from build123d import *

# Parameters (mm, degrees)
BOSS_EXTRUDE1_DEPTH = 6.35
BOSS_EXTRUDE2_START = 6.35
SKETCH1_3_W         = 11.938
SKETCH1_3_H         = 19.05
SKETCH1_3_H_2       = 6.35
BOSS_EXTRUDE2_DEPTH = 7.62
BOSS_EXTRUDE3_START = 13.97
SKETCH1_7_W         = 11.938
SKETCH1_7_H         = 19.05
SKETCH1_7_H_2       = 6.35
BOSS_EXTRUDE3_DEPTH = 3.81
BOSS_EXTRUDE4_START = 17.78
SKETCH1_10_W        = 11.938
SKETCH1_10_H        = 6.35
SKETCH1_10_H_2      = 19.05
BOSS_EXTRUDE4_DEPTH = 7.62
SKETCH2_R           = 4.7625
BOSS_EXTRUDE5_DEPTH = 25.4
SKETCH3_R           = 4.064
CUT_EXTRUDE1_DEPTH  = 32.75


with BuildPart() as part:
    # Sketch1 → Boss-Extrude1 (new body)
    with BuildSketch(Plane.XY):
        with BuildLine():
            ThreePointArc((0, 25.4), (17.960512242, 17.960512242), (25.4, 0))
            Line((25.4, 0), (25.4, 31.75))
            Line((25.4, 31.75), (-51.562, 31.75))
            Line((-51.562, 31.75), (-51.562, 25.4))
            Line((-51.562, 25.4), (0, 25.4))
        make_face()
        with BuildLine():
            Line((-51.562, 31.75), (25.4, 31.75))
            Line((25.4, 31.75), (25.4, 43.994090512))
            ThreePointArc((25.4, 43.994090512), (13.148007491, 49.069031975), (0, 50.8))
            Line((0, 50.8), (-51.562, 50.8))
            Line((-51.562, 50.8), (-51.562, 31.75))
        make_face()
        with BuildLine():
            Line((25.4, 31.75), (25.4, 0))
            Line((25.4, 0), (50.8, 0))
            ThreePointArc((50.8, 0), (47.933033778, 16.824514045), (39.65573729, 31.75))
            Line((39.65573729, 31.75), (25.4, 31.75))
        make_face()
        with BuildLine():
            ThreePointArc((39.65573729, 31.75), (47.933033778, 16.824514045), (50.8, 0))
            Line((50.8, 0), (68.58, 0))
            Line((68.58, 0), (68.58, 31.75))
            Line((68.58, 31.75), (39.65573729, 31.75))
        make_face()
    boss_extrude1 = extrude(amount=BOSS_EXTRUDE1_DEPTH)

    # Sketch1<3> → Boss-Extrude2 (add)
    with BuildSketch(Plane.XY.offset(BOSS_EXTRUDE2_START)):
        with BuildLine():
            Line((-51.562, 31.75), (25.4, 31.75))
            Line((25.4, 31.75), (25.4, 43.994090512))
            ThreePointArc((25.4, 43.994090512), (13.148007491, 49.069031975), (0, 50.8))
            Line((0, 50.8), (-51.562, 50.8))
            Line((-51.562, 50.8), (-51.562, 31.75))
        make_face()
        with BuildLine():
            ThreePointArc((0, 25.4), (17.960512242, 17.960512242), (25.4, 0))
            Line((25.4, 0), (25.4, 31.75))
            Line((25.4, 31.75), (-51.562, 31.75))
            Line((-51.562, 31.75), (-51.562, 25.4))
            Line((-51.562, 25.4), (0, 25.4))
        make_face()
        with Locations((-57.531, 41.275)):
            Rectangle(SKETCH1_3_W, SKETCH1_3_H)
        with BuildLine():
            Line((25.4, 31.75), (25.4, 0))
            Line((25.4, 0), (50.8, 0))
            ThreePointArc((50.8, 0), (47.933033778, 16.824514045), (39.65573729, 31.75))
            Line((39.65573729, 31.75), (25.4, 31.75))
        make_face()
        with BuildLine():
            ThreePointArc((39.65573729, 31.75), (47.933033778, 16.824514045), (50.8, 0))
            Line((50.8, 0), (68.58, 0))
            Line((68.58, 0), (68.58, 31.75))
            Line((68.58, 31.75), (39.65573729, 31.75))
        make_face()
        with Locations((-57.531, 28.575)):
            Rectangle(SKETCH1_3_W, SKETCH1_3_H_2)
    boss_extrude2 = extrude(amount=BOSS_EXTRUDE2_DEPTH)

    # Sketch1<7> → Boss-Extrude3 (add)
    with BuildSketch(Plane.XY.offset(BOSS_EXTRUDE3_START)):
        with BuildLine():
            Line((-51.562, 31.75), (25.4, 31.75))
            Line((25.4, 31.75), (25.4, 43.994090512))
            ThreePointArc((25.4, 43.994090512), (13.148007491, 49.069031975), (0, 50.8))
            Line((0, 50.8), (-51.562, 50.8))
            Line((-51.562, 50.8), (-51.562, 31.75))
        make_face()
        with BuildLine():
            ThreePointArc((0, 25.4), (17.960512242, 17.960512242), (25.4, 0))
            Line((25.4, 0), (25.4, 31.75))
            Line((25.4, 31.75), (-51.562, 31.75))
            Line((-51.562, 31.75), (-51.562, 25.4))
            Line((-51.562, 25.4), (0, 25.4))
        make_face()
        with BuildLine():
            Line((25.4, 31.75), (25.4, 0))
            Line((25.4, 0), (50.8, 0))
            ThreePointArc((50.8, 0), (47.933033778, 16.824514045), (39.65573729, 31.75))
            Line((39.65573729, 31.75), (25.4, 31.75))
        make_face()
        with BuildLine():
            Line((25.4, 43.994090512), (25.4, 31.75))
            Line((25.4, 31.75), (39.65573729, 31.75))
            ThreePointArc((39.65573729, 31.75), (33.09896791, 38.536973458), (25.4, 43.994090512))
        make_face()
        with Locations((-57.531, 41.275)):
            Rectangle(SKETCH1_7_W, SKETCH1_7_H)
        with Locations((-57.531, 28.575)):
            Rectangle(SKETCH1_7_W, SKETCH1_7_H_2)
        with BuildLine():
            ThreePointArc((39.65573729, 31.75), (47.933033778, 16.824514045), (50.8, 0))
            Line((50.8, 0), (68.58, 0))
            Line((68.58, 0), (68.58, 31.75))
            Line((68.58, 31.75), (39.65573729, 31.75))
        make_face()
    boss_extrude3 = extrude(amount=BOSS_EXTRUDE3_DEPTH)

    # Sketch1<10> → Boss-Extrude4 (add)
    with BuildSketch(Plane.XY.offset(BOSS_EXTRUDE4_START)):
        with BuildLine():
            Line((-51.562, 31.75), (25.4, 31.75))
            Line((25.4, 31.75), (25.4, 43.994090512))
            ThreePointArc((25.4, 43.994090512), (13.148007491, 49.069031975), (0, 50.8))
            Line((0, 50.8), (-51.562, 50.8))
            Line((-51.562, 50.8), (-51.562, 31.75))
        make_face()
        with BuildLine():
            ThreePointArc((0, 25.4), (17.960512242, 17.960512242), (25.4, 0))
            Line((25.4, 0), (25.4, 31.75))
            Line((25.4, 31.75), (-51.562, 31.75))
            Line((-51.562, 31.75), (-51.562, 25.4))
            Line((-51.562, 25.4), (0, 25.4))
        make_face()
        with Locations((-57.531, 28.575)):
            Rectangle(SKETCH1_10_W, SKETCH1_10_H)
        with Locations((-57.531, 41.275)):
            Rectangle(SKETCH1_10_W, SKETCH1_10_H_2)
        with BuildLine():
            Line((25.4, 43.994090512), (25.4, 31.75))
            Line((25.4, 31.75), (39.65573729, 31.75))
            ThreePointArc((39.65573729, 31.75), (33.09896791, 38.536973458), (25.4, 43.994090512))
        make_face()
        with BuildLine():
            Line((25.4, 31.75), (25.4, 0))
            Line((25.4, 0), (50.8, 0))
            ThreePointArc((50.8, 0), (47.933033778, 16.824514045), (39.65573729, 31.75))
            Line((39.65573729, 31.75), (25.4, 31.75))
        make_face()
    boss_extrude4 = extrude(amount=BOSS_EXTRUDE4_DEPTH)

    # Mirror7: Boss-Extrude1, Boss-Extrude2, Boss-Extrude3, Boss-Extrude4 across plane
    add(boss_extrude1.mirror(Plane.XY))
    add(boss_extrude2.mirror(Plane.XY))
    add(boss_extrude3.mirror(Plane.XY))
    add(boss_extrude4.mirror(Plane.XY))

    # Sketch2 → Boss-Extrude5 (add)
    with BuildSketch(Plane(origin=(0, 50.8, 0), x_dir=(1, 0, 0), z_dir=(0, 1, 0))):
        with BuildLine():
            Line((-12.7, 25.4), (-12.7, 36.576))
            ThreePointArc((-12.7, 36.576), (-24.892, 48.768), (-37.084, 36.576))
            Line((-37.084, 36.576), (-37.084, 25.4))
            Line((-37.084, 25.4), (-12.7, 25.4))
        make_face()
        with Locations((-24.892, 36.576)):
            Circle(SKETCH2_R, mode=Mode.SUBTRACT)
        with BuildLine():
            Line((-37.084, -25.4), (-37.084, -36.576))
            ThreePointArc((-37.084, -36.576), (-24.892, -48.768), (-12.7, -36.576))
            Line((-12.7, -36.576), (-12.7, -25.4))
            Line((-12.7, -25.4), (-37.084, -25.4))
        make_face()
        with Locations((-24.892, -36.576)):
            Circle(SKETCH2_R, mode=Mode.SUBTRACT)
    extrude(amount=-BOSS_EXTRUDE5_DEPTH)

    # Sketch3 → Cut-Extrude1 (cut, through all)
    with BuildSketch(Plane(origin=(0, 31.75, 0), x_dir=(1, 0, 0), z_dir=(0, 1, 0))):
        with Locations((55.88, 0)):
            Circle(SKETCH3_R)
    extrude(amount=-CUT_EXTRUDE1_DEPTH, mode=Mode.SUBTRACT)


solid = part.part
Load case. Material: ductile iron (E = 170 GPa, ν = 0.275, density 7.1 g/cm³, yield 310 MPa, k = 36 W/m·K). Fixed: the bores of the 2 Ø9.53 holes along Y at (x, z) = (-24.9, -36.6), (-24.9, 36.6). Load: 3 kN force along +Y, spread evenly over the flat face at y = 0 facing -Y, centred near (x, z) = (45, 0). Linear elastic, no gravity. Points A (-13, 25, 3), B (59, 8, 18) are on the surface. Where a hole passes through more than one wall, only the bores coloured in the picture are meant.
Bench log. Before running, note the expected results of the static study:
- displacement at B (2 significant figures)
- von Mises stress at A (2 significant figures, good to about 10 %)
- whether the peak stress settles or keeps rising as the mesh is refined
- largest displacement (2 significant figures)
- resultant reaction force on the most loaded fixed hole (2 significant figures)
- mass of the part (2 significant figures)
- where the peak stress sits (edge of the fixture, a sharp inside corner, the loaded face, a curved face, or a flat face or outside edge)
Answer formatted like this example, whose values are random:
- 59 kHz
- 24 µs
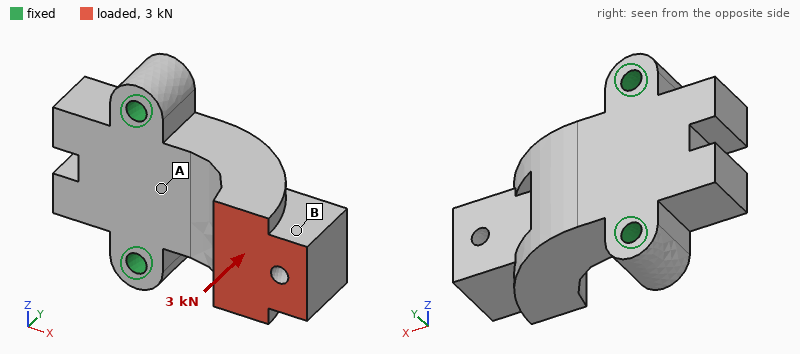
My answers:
- 76 µm
- 23 MPa
- keeps rising
- 89 µm
- 1.5 kN
- 1.4 kg
- edge of the fixture
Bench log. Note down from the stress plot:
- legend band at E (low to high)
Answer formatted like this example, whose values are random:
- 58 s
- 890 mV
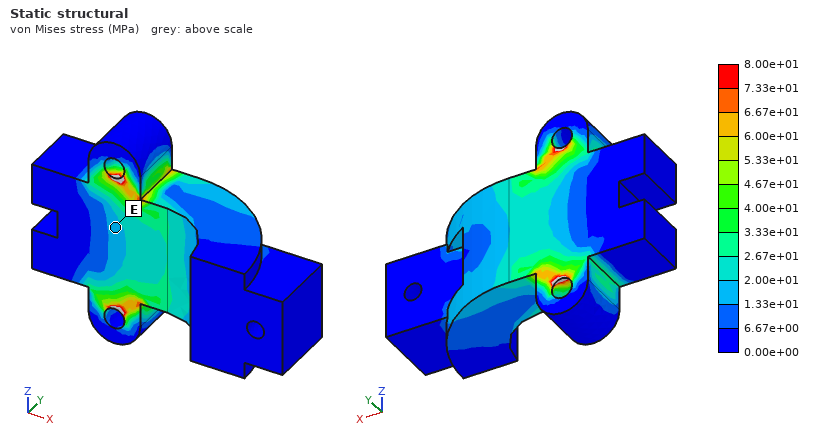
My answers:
- 1.33e+01 to 2.00e+01 MPa
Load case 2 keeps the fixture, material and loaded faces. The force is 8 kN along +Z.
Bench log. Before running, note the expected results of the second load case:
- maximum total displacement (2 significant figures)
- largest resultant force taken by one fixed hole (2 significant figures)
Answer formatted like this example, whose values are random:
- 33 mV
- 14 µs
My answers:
- 72 µm
- 11 kN
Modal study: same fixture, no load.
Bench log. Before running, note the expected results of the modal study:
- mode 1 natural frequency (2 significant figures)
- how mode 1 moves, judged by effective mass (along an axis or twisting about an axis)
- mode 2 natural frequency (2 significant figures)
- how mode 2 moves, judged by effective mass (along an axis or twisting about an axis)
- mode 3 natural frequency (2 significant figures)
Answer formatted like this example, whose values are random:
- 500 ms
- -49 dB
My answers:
- 1500 Hz
- along Y
- 3300 Hz
- along Z
- 6100 Hz
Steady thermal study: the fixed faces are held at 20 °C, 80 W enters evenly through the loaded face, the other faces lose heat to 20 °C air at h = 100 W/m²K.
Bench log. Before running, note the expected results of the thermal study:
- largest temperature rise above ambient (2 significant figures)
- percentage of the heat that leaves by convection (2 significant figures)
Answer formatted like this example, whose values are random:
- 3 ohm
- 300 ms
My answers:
- 71 K
- 76 %
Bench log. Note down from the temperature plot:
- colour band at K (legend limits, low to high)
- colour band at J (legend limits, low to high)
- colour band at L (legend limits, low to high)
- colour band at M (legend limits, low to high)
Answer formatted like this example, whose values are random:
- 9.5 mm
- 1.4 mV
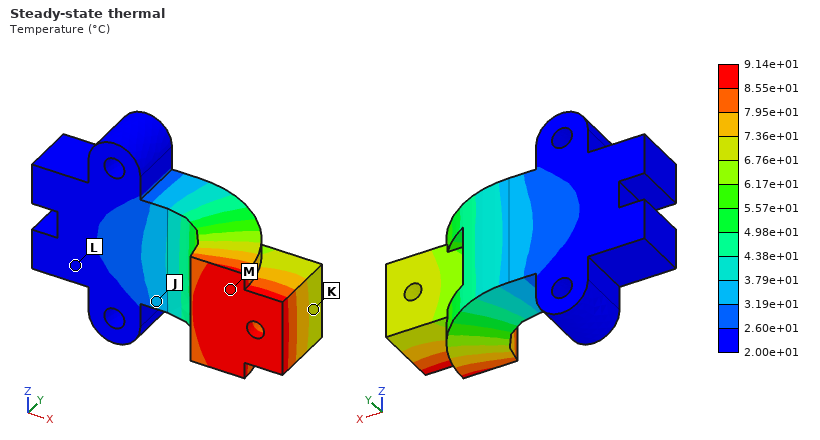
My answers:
- 6.76e+01 to 7.36e+01 °C
- 3.19e+01 to 3.79e+01 °C
- 2.00e+01 to 2.60e+01 °C
- 8.55e+01 to 9.14e+01 °C
